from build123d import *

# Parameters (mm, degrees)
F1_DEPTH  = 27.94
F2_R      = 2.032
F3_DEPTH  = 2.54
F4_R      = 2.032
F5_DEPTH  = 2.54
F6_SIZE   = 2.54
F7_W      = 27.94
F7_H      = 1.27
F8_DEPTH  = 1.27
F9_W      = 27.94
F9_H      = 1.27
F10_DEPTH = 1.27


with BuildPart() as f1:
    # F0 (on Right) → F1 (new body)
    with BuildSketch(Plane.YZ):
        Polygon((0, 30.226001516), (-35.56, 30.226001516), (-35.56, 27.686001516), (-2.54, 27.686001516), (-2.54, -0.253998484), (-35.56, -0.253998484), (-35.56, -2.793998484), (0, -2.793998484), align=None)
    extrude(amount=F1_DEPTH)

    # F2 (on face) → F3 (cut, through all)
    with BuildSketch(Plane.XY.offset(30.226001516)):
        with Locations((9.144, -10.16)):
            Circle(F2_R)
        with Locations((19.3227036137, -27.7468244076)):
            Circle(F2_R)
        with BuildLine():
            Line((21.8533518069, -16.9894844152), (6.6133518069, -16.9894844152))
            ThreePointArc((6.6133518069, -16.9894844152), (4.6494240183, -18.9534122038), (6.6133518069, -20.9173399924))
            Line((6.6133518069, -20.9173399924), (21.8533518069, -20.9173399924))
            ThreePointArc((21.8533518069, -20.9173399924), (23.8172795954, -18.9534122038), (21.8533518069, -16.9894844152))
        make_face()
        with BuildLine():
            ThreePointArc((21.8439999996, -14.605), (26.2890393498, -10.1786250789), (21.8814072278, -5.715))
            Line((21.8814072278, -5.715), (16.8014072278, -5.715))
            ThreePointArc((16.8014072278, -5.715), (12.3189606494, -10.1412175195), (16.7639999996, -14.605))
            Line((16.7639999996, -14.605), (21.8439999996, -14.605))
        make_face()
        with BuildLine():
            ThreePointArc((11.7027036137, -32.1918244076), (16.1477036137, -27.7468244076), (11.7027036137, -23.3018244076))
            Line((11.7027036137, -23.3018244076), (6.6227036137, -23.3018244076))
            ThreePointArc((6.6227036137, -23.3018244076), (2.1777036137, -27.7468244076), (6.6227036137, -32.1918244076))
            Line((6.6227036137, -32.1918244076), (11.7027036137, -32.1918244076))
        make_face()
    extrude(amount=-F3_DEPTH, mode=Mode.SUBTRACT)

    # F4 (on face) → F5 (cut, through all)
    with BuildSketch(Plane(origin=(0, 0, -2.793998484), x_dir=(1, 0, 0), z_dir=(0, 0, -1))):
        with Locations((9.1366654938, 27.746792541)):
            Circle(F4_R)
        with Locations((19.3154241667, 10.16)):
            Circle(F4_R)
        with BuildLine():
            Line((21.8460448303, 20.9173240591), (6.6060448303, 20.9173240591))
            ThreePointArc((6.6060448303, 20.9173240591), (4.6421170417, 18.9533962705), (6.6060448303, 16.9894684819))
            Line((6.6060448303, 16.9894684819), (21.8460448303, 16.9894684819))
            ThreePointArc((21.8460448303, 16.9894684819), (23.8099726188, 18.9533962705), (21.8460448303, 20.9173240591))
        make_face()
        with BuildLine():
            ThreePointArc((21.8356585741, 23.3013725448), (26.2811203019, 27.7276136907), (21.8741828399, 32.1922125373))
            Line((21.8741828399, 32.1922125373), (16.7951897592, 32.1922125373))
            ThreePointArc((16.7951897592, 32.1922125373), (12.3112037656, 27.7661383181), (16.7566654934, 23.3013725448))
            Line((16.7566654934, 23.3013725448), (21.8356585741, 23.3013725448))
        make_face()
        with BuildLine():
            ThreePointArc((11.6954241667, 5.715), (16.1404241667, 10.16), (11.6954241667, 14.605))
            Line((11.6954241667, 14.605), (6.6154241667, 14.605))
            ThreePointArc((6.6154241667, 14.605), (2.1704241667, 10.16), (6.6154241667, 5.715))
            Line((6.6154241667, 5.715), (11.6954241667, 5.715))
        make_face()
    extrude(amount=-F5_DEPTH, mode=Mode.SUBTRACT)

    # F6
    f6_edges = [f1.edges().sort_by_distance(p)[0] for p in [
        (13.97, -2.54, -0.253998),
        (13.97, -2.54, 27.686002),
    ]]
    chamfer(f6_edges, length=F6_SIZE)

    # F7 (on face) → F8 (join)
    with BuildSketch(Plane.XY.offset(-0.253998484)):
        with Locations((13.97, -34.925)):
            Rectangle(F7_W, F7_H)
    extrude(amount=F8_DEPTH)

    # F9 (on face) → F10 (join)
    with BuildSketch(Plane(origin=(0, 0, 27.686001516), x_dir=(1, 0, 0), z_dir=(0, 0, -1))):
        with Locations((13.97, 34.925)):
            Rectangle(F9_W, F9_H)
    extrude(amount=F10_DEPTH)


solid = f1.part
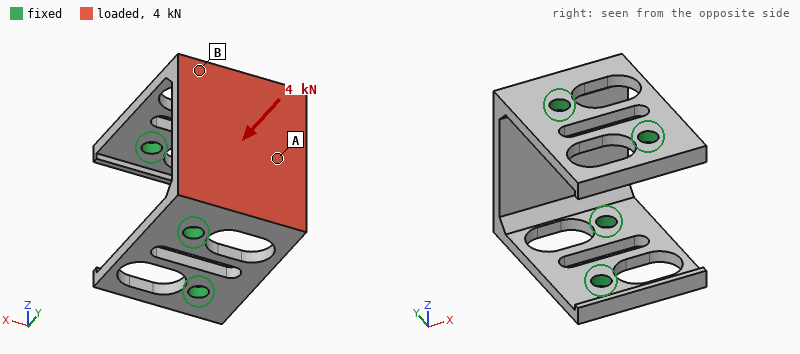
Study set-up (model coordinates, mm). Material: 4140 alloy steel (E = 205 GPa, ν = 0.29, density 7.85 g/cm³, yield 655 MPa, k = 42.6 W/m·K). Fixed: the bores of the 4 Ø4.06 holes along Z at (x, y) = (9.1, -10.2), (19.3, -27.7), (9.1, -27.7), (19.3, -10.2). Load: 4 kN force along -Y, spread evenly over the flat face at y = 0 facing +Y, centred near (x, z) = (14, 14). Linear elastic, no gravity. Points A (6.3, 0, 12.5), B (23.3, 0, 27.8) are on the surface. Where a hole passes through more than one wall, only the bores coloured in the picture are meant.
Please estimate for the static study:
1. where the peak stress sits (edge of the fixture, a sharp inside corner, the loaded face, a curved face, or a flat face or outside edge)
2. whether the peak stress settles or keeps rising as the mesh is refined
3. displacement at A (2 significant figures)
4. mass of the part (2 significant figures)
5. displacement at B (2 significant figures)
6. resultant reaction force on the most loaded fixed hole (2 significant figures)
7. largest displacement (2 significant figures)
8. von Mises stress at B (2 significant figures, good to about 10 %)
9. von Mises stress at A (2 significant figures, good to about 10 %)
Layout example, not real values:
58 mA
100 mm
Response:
edge of the fixture
keeps rising
44 µm
45 g
11 µm
2.2 kN
50 µm
42 MPa
170 MPa
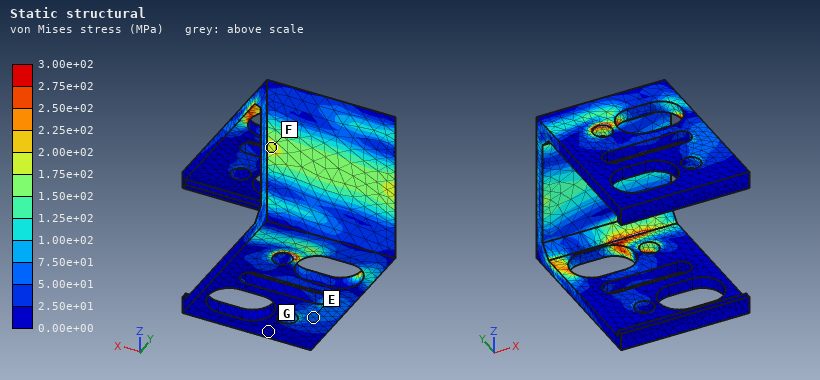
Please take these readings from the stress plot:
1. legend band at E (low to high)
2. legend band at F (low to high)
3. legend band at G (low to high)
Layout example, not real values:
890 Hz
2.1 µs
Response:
5.00e+01 to 7.50e+01 MPa
1.75e+02 to 2.00e+02 MPa
0.00e+00 to 2.50e+01 MPa
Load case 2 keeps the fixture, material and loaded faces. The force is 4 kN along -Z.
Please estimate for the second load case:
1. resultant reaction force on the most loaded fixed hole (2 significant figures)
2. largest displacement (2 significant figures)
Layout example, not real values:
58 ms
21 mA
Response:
2.1 kN
45 µm
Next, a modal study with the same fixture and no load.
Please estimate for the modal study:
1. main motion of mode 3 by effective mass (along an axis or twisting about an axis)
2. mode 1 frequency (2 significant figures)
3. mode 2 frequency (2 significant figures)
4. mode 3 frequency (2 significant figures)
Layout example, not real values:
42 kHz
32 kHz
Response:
along Z
7400 Hz
7700 Hz
11 kHz
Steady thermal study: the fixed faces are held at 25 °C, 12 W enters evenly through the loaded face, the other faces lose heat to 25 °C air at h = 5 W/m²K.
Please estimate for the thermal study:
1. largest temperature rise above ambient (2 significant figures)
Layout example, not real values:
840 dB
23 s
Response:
41 K
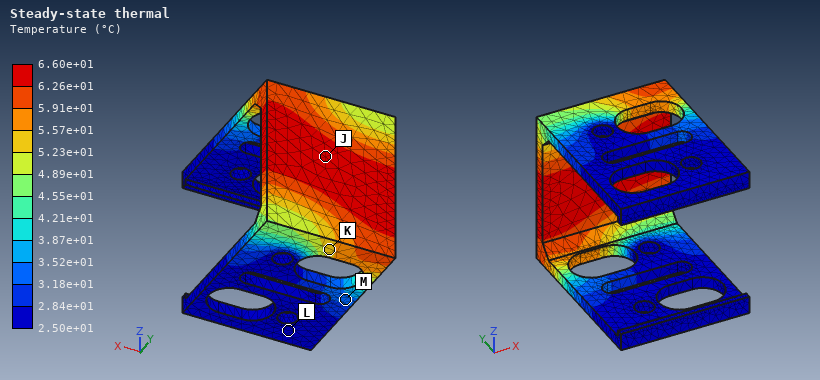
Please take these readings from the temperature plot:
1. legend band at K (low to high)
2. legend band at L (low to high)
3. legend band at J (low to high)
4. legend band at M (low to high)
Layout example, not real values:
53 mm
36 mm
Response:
5.23e+01 to 5.57e+01 °C
2.50e+01 to 2.84e+01 °C
6.26e+01 to 6.60e+01 °C
3.18e+01 to 3.52e+01 °C
